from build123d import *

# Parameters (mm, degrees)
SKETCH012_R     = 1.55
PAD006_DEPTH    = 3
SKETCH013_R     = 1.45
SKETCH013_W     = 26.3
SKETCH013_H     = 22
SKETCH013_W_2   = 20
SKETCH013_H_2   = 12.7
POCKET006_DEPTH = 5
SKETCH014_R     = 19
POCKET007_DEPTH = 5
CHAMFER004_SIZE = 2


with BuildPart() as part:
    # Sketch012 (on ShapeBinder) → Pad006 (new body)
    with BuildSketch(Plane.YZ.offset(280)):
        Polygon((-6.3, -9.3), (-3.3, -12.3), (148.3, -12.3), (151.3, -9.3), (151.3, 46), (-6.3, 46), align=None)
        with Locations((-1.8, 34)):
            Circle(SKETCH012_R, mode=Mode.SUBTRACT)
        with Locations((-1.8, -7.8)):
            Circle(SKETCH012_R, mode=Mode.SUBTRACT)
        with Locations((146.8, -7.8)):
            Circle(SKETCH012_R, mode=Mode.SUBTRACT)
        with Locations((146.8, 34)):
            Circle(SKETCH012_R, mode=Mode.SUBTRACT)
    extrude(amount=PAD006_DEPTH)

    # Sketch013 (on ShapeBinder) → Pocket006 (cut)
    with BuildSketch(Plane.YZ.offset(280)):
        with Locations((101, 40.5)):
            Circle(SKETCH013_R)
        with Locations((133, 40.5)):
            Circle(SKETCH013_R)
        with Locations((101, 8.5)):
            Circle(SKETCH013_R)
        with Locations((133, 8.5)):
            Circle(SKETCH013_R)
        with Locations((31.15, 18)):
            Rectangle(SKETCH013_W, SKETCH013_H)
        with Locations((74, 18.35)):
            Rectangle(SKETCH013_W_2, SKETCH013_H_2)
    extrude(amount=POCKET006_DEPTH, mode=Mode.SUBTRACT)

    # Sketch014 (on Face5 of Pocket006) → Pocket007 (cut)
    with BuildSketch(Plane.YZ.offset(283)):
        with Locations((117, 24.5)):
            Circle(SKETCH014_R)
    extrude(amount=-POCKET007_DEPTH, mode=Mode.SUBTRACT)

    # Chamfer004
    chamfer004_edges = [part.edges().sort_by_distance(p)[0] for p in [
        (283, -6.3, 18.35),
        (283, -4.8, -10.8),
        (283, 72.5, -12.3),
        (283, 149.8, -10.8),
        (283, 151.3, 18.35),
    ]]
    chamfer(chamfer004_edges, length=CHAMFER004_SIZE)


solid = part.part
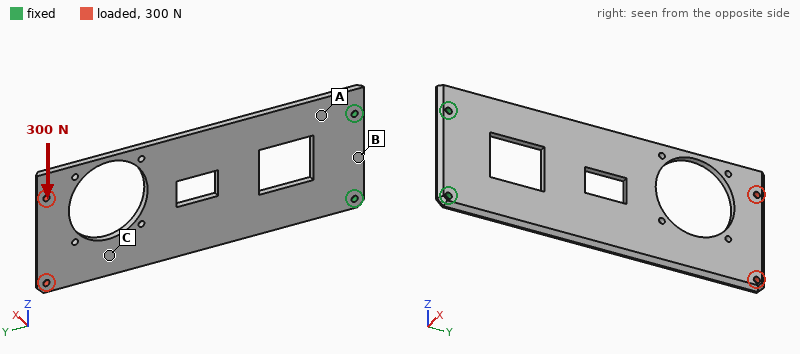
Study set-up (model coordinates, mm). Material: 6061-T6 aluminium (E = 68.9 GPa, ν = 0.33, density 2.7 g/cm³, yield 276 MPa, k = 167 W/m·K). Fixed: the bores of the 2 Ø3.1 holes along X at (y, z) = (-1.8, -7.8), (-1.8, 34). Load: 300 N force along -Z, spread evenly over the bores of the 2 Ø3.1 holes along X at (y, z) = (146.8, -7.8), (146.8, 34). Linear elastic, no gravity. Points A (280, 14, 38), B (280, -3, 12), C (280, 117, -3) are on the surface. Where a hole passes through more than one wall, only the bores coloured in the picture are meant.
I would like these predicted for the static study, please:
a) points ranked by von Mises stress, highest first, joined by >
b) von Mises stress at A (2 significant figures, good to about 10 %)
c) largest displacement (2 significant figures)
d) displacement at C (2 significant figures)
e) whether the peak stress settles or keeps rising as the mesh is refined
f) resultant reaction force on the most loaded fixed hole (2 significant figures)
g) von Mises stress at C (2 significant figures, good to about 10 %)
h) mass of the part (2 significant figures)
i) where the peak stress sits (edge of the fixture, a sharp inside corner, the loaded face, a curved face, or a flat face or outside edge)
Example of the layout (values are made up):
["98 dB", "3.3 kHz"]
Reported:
["A > C > B", "22 MPa", "0.22 mm", "0.14 mm", "keeps rising", "1.1 kN", "13 MPa", "57 g", "edge of the fixture"]
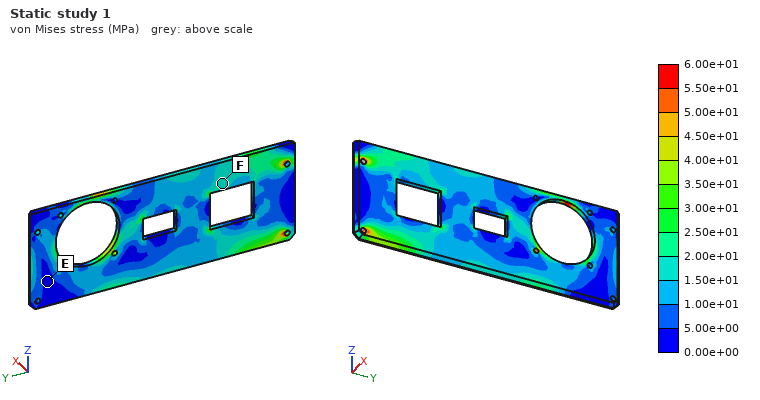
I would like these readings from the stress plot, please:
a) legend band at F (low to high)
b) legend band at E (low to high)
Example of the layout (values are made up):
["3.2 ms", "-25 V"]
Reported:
["1.50e+01 to 2.00e+01 MPa", "0.00e+00 to 5.00e+00 MPa"]
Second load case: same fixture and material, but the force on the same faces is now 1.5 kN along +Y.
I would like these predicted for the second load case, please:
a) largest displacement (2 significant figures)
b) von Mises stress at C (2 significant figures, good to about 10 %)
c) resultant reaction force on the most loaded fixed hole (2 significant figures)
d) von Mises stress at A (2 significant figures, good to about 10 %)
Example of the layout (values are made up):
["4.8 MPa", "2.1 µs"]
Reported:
["72 µm", "18 MPa", "770 N", "12 MPa"]
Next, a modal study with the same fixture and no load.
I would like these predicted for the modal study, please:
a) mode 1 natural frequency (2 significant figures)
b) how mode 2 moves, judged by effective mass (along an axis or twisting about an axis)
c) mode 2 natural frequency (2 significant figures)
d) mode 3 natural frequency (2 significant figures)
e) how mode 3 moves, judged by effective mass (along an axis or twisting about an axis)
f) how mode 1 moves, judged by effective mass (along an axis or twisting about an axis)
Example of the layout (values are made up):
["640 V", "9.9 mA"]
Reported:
["100 Hz", "twisting about Y", "530 Hz", "570 Hz", "along X", "along X"]
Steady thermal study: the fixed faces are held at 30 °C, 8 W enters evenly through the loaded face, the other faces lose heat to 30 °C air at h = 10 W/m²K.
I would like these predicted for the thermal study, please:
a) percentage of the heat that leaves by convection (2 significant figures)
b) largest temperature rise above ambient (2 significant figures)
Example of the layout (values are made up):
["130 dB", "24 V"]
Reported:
["42 %", "56 K"]
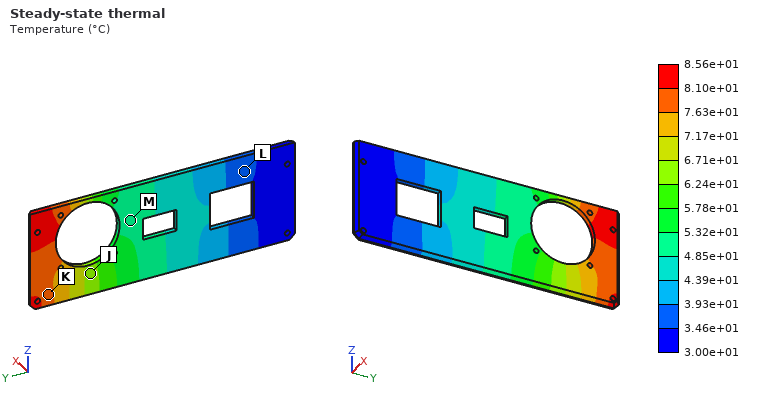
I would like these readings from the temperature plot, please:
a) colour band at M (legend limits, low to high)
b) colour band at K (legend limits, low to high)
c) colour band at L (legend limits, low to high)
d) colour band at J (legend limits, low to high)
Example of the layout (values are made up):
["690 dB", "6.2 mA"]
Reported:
["4.85e+01 to 5.32e+01 °C", "7.63e+01 to 8.10e+01 °C", "3.46e+01 to 3.93e+01 °C", "6.24e+01 to 6.71e+01 °C"]
